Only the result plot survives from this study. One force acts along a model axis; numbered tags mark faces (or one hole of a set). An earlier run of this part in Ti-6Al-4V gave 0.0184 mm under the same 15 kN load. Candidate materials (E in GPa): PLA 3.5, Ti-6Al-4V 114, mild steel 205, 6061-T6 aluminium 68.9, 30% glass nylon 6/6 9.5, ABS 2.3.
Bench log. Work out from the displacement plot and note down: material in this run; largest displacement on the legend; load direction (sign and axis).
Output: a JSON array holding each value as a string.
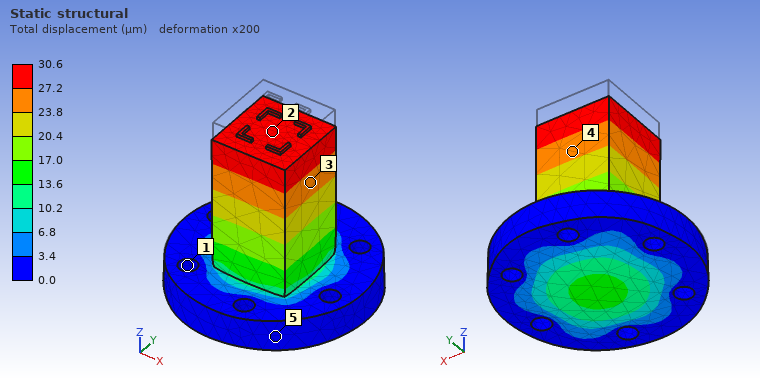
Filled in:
["6061-T6 aluminium", "30.6 µm", "-Z"]
